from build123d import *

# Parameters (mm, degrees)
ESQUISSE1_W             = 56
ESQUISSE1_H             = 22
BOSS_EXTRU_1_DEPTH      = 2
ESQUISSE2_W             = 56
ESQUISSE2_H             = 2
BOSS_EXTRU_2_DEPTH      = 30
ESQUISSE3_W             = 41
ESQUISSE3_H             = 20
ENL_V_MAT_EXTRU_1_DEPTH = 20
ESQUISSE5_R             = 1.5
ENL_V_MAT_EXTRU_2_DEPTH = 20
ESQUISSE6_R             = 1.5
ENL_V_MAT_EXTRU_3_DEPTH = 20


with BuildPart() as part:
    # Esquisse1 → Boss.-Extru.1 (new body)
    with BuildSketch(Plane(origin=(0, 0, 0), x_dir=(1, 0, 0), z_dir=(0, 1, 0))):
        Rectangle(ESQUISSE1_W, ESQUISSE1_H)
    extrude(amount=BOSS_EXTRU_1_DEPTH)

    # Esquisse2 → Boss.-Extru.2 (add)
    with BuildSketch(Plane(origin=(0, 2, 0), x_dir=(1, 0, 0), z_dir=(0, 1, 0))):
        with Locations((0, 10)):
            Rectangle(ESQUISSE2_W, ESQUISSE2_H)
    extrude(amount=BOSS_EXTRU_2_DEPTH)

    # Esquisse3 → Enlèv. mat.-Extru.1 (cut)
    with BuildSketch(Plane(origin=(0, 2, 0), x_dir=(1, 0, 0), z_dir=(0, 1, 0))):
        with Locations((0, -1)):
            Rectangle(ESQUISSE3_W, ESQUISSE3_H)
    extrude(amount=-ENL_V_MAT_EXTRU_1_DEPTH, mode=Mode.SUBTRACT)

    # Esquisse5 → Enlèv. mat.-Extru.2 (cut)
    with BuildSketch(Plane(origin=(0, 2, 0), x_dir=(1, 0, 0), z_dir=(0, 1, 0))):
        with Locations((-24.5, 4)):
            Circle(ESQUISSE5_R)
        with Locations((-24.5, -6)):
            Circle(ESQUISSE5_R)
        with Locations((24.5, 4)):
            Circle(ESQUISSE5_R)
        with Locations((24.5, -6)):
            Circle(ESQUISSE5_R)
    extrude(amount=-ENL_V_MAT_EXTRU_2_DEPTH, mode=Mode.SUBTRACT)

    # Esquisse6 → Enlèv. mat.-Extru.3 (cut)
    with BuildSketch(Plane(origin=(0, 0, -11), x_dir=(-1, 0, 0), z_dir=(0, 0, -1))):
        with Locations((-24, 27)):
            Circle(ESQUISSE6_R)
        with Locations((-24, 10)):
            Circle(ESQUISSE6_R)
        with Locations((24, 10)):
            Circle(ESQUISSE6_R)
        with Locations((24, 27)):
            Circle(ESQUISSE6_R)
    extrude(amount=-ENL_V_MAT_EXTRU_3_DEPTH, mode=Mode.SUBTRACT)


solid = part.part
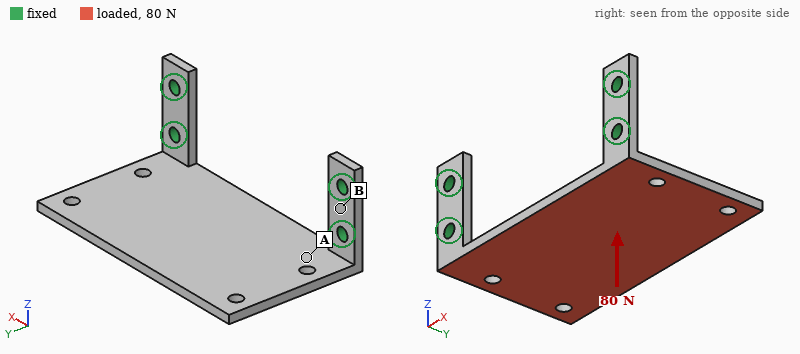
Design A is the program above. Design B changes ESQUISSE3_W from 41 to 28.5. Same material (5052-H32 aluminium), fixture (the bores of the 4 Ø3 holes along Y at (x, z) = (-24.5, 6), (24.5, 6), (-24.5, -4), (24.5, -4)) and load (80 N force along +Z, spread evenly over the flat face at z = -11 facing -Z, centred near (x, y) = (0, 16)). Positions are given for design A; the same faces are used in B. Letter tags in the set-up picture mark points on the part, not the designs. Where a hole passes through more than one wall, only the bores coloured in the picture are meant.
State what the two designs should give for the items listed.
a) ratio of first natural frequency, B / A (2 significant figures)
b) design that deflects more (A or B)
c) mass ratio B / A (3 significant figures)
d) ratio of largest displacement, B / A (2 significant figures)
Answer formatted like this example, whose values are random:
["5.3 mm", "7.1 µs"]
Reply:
["1.2", "A", "1.12", "0.65"]
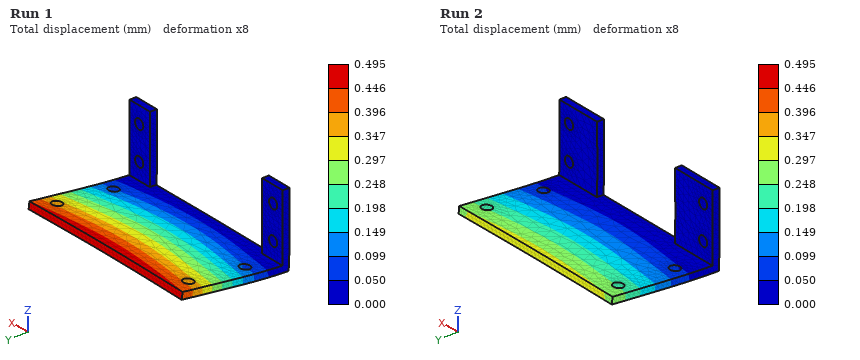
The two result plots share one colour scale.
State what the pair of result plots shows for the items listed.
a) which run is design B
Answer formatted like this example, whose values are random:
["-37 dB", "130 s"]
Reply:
["Run 2"]
